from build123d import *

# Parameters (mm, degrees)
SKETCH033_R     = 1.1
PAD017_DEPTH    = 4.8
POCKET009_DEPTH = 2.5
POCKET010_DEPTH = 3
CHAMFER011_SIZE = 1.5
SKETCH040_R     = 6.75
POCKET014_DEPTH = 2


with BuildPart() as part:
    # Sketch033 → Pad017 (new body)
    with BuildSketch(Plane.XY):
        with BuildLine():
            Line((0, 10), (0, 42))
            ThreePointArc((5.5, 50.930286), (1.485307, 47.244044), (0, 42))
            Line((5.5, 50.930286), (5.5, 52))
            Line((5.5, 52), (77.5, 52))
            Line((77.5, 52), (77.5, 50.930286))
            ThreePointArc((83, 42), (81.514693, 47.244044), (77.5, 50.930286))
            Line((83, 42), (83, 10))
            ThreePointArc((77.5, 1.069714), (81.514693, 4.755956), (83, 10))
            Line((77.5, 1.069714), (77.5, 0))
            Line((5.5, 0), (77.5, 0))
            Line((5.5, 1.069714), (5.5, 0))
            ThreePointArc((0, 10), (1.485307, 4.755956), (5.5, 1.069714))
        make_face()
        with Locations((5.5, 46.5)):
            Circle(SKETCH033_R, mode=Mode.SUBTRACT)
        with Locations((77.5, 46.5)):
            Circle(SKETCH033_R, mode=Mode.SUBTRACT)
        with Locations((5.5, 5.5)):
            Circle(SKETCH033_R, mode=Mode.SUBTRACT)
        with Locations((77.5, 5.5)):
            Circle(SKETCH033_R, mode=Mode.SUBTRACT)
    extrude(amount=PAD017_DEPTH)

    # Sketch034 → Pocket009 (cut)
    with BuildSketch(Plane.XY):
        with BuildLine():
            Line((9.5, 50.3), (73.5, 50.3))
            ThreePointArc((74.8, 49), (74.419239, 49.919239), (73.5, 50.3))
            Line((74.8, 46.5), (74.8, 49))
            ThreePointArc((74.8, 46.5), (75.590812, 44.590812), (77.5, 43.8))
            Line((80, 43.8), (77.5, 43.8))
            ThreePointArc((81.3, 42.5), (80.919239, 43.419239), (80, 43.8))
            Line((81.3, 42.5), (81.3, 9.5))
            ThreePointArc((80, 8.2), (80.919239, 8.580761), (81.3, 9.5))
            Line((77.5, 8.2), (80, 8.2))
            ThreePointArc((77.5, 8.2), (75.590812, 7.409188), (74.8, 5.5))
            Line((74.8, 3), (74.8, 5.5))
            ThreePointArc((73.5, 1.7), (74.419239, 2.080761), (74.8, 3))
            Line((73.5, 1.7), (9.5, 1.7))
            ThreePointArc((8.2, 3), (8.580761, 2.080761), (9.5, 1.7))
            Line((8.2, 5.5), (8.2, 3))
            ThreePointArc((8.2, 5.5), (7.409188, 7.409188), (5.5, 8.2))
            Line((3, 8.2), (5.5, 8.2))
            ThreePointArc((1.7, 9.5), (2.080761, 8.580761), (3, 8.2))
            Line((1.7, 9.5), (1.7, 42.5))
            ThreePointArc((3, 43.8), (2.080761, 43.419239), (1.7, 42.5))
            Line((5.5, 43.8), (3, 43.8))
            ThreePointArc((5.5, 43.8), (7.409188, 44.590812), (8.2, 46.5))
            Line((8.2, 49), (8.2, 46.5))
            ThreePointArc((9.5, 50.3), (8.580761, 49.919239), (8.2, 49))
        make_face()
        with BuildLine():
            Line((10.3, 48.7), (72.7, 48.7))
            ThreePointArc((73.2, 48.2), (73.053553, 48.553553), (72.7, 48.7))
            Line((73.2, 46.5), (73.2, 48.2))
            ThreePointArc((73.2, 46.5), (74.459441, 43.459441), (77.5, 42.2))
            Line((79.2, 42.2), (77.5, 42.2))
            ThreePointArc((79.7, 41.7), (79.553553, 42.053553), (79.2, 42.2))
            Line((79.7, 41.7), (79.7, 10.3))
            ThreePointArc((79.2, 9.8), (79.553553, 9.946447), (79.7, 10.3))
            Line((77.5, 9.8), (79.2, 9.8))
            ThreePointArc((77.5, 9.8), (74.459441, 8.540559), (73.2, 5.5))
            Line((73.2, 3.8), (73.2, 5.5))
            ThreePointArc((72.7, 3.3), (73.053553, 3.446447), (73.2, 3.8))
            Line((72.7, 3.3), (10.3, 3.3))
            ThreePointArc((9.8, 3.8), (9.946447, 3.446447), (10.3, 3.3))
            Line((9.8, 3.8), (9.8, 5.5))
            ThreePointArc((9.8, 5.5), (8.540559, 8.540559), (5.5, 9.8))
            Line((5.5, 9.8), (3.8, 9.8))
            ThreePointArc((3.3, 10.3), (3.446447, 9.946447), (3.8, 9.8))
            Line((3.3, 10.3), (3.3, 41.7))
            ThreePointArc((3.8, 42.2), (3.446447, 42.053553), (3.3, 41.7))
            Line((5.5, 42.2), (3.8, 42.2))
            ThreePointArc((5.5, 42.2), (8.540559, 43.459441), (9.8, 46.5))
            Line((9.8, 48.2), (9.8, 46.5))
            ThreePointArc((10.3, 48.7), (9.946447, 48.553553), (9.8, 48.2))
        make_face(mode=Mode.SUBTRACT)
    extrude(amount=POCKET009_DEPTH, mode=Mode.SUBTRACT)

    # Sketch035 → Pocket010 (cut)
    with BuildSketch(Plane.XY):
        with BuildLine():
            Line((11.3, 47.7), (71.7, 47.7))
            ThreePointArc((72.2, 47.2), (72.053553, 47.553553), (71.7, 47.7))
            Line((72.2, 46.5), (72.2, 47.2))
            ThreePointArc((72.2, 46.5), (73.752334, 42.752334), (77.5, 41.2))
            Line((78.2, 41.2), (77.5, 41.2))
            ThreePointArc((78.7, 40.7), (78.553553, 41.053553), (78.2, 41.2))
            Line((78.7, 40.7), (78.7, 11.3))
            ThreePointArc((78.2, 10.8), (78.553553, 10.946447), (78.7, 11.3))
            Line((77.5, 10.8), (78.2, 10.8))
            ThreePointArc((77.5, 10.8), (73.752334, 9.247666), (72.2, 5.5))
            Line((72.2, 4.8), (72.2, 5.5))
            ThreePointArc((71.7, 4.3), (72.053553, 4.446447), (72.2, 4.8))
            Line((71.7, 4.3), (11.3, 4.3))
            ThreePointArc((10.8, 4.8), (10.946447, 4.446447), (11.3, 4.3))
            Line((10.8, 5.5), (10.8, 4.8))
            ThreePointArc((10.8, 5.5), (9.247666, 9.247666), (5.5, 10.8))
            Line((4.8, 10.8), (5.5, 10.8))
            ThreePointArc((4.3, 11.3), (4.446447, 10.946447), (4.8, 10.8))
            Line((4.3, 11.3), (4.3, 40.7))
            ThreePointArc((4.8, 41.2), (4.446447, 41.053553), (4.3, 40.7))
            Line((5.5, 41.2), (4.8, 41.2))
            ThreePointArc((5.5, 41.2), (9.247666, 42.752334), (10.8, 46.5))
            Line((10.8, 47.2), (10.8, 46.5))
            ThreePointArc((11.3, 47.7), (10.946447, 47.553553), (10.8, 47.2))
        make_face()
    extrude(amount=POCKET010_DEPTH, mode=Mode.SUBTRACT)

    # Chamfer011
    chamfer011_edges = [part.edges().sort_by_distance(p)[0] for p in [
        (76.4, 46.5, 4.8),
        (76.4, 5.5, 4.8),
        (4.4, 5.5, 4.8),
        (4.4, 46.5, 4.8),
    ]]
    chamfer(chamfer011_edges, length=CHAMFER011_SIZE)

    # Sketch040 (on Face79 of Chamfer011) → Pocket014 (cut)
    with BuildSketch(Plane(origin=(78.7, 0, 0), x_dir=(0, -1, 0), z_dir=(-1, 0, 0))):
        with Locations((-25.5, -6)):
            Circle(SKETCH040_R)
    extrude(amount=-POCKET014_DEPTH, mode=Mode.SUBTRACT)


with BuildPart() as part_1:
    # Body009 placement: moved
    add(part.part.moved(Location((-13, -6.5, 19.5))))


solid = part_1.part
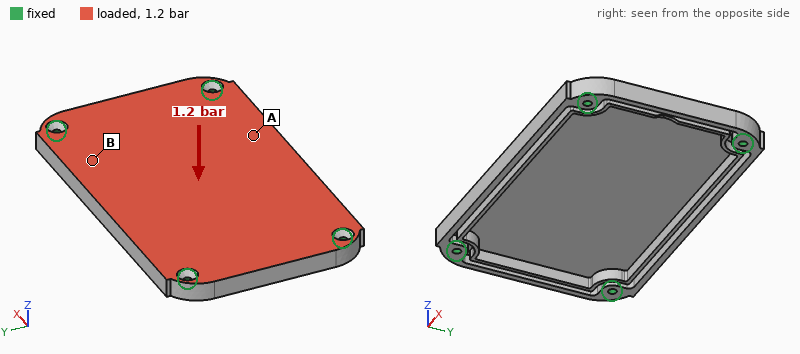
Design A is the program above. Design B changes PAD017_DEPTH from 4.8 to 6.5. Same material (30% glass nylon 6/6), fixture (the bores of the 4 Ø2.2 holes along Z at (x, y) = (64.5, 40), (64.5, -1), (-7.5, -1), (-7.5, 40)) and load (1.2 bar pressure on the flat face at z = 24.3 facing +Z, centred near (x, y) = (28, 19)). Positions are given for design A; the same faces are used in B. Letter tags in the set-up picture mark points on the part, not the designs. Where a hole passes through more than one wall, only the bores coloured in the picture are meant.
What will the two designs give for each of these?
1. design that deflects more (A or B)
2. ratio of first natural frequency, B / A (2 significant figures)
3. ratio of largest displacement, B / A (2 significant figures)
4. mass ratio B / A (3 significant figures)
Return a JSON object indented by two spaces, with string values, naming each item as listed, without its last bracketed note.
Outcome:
{
  "design that deflects more": "A",
  "ratio of first natural frequency, B / A": "1.4",
  "ratio of largest displacement, B / A": "0.23",
  "mass ratio B / A": "1.72"
}
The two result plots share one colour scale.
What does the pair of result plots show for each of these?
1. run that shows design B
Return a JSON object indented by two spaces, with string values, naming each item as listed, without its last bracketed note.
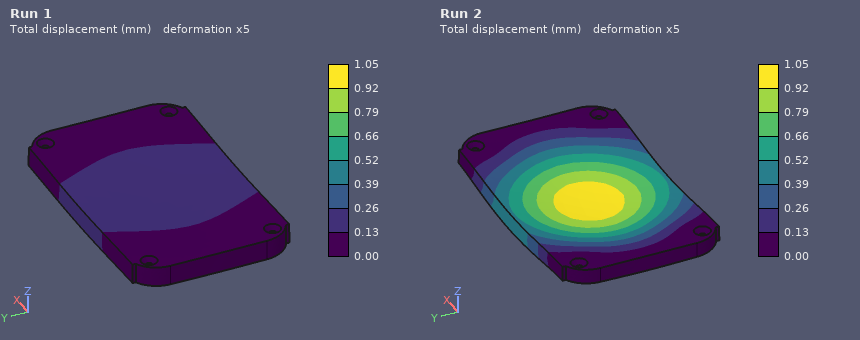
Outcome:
{
  "run that shows design B": "Run 1"
}
